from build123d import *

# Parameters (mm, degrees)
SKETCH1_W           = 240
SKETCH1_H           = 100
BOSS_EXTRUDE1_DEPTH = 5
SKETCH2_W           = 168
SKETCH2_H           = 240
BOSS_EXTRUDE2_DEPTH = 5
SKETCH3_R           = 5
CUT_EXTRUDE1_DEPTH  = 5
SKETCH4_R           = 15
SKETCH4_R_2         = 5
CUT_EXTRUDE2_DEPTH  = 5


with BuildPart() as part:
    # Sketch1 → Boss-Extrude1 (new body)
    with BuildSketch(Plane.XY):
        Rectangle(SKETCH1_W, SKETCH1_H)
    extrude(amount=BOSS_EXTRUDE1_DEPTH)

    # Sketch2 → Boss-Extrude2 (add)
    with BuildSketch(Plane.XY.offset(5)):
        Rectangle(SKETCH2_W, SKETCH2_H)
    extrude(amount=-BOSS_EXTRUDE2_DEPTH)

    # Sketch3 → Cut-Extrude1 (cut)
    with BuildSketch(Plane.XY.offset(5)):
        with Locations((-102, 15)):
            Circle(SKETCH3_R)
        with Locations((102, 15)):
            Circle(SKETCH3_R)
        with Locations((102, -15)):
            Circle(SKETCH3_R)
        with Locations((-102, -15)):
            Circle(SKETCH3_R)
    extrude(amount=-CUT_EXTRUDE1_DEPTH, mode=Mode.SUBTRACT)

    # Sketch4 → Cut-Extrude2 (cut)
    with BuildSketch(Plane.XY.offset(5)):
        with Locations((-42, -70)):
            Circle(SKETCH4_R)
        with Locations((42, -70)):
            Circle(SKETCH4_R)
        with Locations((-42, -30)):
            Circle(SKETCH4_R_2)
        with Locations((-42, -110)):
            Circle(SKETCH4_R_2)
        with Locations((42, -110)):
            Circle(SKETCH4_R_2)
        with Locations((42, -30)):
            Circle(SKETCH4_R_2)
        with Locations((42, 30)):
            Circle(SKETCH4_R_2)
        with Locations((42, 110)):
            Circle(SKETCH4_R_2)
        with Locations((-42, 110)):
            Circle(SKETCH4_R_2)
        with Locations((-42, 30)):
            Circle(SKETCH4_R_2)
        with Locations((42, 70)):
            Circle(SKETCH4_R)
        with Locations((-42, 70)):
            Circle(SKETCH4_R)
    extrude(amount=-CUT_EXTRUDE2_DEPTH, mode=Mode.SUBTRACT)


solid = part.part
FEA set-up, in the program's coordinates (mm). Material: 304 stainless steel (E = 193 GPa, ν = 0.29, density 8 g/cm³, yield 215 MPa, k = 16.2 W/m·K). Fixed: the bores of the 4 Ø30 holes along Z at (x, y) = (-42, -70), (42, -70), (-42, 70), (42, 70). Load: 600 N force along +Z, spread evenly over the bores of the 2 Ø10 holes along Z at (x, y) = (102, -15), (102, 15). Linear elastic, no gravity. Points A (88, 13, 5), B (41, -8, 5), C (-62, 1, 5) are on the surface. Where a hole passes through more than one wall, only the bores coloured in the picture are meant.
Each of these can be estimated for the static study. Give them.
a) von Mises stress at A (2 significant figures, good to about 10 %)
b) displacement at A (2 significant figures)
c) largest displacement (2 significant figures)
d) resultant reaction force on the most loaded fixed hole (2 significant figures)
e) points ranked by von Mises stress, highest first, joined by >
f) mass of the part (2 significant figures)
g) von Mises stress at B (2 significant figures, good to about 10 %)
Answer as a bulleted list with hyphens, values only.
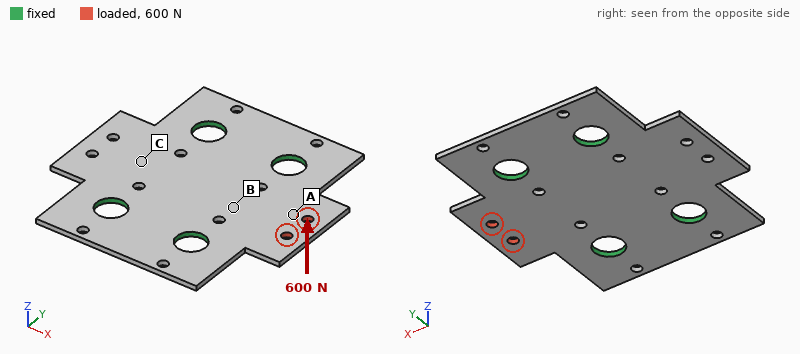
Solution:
- 36 MPa
- 0.13 mm
- 0.27 mm
- 340 N
- A > B > C
- 1.8 kg
- 25 MPa
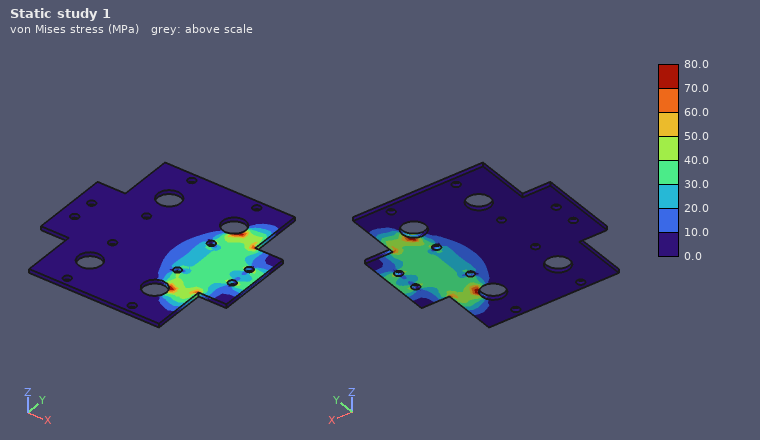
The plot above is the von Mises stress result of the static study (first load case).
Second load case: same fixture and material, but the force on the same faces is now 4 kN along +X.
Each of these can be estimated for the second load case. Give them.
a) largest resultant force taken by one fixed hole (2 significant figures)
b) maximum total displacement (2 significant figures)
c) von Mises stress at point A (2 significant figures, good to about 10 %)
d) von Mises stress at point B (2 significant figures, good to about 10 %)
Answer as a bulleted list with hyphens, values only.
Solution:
- 1.6 kN
- 4.9 µm
- 11 MPa
- 5.2 MPa
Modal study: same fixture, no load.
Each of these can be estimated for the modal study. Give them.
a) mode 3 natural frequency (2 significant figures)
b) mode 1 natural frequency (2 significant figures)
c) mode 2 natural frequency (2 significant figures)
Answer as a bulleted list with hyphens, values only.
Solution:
- 1800 Hz
- 770 Hz
- 770 Hz
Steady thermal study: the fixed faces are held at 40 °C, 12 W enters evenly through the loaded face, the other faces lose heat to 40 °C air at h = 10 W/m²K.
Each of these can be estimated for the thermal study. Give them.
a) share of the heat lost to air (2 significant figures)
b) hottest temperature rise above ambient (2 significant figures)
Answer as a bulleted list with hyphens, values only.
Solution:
- 55 %
- 72 K
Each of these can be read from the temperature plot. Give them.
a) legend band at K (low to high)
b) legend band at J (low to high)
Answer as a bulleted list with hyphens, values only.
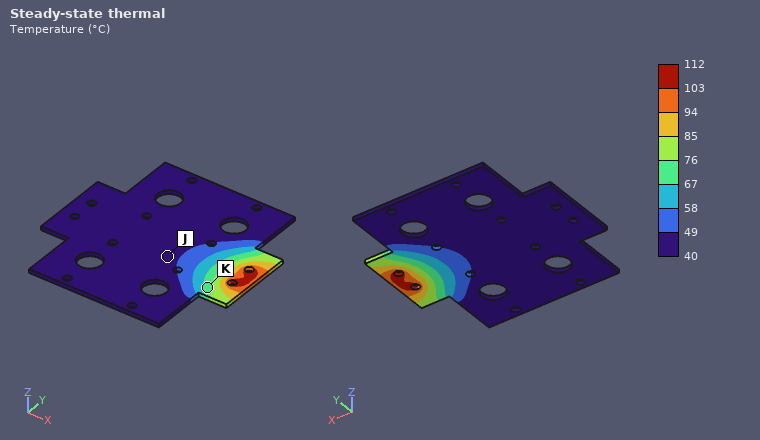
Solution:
- 67 to 76 °C
- 40 to 49 °C
